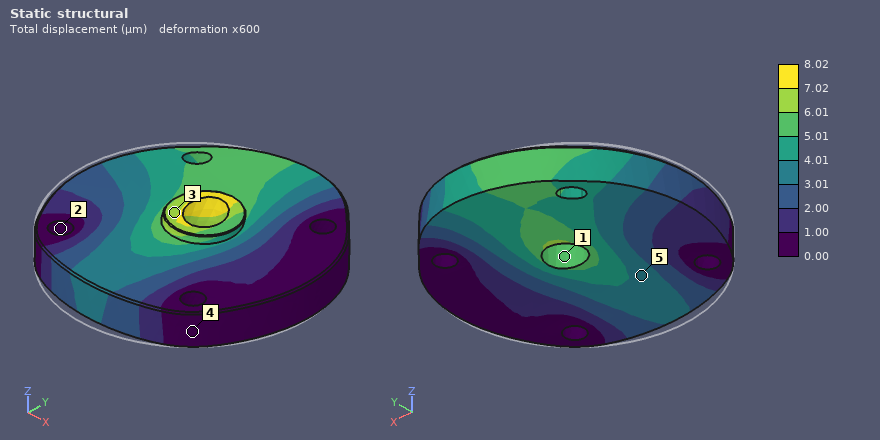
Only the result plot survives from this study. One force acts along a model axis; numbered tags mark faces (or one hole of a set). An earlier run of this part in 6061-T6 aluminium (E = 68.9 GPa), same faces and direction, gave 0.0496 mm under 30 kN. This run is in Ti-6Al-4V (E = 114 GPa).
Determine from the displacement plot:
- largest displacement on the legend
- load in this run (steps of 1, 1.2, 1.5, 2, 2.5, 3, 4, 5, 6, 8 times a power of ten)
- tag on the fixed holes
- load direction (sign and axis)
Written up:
8.02 µm
8 kN
2
+Y
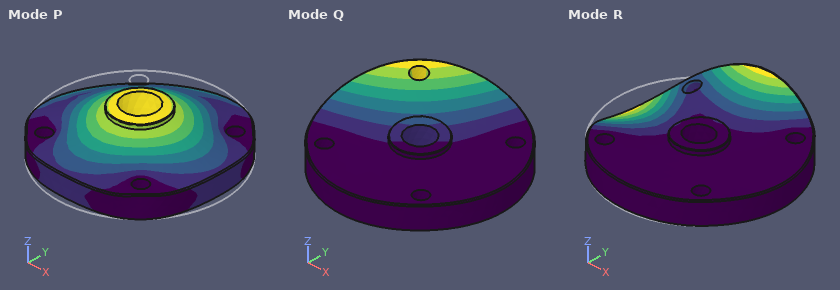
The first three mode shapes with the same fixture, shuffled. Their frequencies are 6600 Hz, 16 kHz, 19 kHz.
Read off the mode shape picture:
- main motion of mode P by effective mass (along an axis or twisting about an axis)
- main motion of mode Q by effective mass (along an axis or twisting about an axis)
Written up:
along Z
along Z
